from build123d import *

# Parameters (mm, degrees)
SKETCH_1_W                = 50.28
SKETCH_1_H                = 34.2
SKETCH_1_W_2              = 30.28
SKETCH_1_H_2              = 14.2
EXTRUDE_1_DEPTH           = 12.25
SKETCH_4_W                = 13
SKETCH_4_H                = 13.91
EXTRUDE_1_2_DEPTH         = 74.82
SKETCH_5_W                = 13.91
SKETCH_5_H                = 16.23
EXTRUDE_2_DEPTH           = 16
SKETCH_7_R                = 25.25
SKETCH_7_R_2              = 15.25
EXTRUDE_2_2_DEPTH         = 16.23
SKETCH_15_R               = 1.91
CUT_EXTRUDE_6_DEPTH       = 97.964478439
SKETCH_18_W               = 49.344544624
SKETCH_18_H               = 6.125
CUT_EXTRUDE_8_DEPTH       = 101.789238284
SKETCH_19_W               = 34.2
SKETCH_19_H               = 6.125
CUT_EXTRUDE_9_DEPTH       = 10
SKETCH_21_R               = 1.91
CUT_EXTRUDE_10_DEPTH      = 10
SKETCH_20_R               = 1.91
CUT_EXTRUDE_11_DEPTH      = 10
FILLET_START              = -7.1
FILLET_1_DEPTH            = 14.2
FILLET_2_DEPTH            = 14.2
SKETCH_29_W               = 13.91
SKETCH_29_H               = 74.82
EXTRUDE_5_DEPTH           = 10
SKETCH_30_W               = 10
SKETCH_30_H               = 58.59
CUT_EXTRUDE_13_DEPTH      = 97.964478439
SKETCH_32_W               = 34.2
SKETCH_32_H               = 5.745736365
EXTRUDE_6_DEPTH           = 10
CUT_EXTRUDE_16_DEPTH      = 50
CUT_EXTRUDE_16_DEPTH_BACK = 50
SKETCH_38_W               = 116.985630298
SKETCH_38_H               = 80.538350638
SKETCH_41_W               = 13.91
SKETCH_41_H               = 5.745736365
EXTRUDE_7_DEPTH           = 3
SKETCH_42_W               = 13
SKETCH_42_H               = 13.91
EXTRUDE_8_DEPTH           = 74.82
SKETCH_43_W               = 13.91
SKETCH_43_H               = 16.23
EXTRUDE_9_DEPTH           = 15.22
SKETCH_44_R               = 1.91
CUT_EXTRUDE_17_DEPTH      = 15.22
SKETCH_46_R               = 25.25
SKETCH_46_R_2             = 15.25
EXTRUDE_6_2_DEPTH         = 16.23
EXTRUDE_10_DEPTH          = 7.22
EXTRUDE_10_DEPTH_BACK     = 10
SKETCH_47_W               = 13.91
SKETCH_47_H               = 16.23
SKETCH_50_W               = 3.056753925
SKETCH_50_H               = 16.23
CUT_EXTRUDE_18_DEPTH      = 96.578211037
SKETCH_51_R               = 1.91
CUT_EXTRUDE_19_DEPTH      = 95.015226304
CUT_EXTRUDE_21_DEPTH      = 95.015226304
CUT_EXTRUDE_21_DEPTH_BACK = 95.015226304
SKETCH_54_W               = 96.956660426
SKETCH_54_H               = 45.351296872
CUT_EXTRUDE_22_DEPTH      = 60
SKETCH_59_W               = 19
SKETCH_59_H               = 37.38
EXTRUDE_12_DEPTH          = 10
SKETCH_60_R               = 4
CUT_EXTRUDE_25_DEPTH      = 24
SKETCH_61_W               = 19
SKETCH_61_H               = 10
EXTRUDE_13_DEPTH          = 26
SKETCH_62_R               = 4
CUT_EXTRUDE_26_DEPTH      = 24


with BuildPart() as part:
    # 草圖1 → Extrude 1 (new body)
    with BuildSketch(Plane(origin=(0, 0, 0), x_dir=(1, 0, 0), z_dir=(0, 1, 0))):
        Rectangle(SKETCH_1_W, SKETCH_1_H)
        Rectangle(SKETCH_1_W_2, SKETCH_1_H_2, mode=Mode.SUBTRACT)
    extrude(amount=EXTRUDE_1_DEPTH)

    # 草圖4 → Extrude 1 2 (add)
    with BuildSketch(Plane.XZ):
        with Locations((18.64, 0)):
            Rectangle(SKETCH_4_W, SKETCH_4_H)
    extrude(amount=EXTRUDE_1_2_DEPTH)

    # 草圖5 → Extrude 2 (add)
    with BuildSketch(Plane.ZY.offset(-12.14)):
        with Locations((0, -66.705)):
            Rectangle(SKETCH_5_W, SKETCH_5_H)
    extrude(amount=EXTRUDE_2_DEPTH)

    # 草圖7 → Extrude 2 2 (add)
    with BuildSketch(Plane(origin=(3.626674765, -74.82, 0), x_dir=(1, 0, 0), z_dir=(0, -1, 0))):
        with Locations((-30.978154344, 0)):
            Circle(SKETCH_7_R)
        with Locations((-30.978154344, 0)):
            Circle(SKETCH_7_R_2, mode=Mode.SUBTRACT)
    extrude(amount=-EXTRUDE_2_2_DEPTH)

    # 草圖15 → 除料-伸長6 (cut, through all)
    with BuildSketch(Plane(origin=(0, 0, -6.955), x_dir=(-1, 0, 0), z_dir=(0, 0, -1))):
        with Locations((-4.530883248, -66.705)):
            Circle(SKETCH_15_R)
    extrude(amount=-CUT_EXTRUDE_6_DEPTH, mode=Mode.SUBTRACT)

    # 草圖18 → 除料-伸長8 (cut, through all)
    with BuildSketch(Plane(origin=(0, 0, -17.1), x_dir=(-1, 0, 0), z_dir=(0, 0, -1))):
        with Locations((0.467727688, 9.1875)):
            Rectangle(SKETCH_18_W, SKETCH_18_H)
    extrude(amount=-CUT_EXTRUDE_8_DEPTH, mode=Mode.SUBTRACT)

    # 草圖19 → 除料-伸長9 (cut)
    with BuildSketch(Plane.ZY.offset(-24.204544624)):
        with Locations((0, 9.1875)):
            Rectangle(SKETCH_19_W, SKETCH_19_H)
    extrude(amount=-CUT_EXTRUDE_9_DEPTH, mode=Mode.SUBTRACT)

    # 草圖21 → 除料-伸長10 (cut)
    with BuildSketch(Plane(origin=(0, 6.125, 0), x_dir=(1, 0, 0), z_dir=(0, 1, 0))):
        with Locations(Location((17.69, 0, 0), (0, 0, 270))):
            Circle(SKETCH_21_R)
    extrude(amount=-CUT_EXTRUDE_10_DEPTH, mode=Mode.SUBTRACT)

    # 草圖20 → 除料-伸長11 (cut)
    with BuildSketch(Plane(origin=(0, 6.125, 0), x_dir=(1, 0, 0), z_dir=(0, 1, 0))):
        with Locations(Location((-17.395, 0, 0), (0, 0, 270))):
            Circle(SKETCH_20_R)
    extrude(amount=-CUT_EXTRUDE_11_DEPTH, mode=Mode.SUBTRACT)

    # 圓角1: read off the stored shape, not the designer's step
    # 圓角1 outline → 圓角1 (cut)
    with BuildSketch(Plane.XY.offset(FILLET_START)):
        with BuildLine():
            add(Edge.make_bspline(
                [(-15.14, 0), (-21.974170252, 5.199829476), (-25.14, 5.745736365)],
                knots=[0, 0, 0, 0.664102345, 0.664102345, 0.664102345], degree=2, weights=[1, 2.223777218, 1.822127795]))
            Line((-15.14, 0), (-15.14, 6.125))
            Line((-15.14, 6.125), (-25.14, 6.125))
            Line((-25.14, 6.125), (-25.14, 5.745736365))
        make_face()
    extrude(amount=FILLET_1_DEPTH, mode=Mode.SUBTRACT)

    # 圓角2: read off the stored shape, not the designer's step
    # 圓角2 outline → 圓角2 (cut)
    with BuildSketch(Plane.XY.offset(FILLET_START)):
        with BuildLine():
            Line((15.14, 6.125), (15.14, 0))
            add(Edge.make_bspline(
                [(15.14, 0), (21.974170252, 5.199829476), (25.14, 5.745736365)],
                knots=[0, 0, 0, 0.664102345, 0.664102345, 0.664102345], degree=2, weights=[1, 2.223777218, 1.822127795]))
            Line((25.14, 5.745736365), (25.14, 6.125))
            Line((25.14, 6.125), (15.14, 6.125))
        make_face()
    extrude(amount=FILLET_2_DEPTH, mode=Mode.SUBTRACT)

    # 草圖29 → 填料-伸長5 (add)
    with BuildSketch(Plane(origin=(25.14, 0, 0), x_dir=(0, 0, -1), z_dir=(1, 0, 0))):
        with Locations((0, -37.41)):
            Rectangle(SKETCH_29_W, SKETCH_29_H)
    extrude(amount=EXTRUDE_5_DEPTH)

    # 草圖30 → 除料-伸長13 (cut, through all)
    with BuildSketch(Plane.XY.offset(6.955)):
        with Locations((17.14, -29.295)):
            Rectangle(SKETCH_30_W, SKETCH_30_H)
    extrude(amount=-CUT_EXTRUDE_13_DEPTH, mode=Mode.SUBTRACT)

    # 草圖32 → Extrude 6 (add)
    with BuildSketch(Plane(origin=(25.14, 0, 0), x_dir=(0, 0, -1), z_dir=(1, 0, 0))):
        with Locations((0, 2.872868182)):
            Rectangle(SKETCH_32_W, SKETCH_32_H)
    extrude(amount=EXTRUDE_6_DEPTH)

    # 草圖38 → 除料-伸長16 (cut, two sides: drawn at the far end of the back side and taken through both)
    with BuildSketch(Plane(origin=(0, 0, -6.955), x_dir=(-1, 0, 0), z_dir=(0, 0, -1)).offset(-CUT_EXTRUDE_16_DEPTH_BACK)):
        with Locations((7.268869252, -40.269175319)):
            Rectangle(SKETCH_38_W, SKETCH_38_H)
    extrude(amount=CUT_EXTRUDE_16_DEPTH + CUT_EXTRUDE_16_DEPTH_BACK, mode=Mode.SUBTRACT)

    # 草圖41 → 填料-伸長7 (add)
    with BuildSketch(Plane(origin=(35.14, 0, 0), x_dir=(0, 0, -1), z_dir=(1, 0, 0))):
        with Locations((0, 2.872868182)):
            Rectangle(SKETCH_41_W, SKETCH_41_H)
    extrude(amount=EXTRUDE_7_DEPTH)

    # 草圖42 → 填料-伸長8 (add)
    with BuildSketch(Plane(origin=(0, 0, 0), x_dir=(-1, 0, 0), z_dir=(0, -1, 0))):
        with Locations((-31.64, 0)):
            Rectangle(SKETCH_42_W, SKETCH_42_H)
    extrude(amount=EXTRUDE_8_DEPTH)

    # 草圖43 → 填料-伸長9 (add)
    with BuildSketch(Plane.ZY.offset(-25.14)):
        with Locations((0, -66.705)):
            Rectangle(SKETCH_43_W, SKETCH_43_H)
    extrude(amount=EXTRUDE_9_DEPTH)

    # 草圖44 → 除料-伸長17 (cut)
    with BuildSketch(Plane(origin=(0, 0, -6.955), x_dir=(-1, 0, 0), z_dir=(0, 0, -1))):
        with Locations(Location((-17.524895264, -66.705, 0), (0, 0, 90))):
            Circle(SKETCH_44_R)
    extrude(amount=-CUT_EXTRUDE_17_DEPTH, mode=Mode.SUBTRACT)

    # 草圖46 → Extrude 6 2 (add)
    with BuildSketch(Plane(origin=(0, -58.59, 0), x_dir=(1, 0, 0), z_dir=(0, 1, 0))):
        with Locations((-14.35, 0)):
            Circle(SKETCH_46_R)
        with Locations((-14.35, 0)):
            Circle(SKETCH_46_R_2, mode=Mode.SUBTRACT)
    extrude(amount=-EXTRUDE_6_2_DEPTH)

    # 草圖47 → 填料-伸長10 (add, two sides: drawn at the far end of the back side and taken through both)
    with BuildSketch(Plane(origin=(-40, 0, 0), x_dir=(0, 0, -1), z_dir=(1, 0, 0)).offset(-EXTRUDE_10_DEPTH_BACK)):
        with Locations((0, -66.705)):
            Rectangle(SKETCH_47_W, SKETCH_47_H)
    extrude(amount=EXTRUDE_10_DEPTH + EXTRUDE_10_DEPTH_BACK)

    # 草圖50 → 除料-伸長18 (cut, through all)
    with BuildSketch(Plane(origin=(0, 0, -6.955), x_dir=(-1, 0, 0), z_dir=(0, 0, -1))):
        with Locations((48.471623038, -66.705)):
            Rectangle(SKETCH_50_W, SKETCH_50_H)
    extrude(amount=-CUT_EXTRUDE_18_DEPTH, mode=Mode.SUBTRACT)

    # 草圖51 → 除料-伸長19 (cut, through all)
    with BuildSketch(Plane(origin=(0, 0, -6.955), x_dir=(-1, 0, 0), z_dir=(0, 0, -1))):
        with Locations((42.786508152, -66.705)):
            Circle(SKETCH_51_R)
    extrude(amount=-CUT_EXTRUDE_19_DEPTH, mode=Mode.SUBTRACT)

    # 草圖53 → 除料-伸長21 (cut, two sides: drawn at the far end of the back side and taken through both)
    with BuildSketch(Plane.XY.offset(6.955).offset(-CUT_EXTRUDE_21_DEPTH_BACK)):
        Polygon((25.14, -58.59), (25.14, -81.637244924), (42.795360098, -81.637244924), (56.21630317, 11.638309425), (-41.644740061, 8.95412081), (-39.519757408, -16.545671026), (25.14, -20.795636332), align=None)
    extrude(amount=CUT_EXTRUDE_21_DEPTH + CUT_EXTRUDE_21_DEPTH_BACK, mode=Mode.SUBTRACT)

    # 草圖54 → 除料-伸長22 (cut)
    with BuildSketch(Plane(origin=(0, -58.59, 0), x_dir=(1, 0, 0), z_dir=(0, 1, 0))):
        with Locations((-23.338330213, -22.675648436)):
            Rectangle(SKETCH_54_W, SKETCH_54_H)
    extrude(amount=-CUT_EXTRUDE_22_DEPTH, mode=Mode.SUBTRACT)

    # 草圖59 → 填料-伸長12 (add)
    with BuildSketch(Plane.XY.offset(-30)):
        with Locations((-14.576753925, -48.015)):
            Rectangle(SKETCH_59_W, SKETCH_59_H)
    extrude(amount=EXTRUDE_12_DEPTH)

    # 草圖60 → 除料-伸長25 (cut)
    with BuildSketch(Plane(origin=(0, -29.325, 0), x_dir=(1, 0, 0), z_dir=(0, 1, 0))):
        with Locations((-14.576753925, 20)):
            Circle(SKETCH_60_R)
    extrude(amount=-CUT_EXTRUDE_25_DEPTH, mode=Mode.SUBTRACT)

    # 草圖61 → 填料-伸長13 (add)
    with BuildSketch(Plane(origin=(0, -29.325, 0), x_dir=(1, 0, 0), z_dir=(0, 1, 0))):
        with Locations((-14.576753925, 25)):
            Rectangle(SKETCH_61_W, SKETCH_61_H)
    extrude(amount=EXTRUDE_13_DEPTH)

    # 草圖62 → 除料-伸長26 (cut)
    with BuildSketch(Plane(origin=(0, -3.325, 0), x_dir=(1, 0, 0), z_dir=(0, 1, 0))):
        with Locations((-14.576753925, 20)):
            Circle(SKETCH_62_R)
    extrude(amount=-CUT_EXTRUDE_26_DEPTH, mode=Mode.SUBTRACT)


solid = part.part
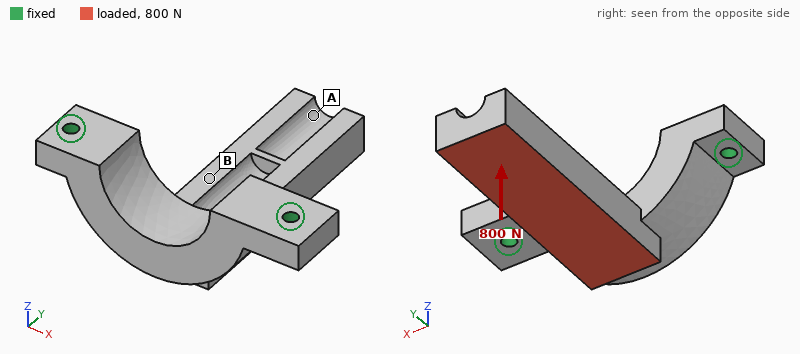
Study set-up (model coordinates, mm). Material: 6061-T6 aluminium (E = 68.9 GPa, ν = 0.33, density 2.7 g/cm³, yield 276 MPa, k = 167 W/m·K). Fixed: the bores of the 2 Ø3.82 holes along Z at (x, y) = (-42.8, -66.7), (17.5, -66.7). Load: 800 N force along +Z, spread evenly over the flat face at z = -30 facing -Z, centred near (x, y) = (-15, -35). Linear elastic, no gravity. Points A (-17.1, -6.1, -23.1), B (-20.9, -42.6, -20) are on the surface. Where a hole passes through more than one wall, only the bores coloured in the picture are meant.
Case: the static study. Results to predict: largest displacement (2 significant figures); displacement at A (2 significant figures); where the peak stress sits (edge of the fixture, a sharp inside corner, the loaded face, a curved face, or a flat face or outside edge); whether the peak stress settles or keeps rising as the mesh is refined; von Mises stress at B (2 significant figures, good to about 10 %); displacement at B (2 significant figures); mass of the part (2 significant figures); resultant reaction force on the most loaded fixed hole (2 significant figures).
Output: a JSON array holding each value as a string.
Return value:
["0.56 mm", "0.52 mm", "edge of the fixture", "keeps rising", "43 MPa", "0.17 mm", "62 g", "610 N"]
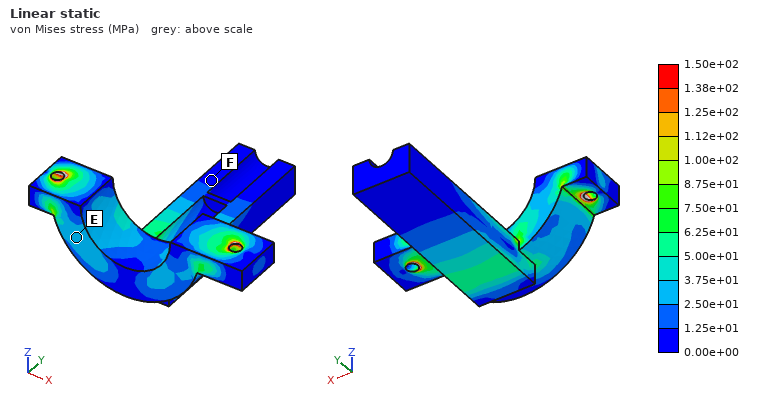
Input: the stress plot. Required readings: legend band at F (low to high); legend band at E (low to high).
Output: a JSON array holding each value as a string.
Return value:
["0.00e+00 to 1.25e+01 MPa", "2.50e+01 to 3.75e+01 MPa"]
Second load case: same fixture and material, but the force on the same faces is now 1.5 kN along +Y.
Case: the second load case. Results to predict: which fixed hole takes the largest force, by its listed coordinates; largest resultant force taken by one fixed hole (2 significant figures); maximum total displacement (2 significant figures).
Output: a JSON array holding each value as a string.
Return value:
["(-42.8, -66.7)", "830 N", "0.55 mm"]
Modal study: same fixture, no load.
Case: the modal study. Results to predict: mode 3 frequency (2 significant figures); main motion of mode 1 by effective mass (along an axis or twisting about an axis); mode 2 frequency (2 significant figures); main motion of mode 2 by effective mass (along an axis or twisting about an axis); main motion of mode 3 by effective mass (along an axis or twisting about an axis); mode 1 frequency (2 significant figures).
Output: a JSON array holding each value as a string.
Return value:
["4000 Hz", "along Z", "2800 Hz", "along X", "along Y", "1300 Hz"]
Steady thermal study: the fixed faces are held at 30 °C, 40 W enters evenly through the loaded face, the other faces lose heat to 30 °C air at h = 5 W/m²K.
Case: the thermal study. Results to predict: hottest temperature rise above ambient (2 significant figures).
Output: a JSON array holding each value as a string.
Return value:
["66 K"]
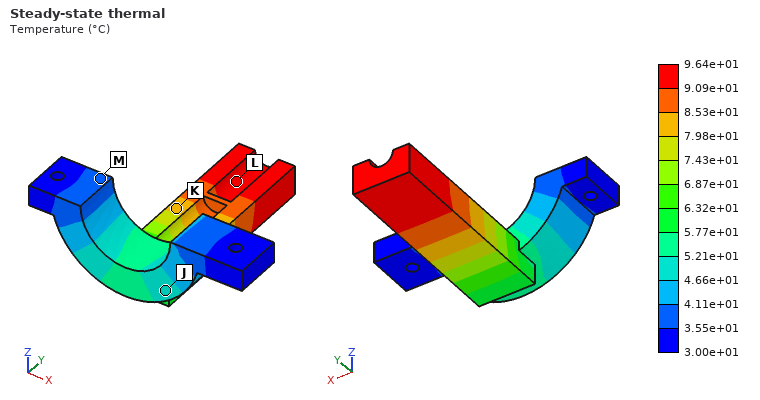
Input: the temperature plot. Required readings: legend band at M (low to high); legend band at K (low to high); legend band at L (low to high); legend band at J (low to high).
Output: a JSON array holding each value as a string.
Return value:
["3.55e+01 to 4.11e+01 °C", "7.98e+01 to 8.53e+01 °C", "9.09e+01 to 9.64e+01 °C", "4.66e+01 to 5.21e+01 °C"]
